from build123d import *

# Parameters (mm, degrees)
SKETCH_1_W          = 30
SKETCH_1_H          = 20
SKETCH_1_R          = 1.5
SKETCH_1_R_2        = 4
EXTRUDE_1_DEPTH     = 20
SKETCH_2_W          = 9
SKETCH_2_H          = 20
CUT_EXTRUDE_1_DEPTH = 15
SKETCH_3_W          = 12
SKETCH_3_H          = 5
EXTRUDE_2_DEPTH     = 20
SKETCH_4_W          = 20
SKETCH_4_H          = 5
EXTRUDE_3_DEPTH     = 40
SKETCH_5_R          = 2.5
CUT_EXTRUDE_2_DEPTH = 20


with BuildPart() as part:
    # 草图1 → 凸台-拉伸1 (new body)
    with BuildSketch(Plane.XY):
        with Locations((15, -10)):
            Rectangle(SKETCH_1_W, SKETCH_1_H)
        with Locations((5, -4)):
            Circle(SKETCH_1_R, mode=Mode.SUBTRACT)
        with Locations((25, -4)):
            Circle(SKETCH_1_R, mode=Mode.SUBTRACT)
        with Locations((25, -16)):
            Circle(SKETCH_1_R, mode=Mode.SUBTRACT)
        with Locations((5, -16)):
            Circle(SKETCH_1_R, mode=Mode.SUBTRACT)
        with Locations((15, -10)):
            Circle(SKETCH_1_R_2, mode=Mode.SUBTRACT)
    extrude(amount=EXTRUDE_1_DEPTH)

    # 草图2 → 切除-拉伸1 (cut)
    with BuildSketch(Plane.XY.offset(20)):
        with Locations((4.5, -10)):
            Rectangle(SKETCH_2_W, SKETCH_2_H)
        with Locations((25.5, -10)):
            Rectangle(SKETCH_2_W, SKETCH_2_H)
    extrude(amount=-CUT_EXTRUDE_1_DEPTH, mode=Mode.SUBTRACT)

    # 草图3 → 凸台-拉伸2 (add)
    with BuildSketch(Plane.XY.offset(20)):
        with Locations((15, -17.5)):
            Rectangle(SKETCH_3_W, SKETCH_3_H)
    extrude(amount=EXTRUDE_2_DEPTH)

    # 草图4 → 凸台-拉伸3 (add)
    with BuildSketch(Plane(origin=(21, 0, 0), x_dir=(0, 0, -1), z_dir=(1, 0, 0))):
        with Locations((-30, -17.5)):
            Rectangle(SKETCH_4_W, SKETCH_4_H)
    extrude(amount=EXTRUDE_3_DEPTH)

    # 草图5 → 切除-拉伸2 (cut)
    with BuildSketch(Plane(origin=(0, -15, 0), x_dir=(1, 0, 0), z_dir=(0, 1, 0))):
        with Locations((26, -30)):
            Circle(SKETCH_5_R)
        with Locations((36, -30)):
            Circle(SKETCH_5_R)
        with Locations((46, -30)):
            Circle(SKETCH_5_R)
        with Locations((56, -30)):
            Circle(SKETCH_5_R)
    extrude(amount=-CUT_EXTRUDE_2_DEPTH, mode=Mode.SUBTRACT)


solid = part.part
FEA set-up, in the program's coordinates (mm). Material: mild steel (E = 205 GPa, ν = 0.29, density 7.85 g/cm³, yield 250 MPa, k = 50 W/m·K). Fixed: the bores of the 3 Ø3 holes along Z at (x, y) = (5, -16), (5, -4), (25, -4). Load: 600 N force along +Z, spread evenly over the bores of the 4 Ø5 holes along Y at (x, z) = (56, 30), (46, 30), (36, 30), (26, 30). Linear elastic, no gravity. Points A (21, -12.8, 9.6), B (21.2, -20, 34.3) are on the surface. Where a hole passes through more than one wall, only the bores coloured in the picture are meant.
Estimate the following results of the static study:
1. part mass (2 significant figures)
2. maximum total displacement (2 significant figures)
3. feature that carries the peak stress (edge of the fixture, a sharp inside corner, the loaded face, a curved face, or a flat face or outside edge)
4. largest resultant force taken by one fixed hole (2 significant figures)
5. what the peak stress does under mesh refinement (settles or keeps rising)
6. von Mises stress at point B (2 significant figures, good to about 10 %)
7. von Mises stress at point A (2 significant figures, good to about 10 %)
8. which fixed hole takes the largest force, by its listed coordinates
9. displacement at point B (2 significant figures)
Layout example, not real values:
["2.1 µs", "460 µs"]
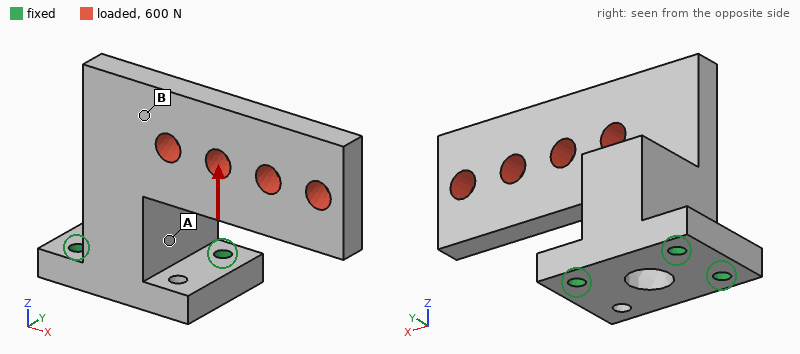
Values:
["81 g", "0.13 mm", "edge of the fixture", "1.2 kN", "keeps rising", "21 MPa", "55 MPa", "(25, -4)", "0.048 mm"]
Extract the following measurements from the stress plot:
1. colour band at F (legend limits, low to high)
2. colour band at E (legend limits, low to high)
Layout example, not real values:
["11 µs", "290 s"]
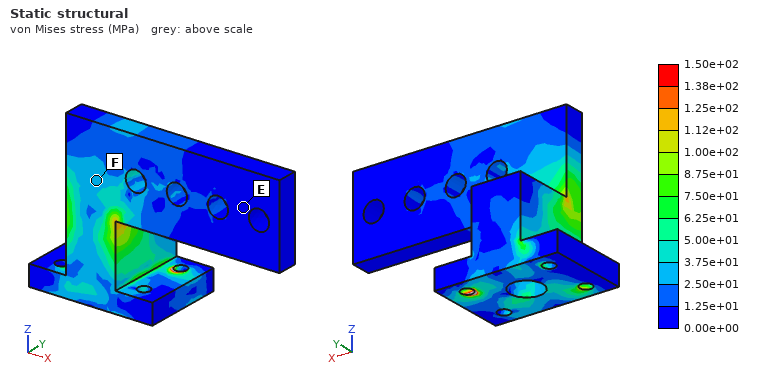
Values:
["2.50e+01 to 3.75e+01 MPa", "0.00e+00 to 1.25e+01 MPa"]
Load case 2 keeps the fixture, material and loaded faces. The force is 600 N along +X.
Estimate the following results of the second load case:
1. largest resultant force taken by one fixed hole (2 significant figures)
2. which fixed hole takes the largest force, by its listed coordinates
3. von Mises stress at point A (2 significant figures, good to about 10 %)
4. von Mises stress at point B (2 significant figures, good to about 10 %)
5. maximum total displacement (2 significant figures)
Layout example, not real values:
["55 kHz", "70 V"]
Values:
["1.0 kN", "(25, -4)", "44 MPa", "9.0 MPa", "69 µm"]
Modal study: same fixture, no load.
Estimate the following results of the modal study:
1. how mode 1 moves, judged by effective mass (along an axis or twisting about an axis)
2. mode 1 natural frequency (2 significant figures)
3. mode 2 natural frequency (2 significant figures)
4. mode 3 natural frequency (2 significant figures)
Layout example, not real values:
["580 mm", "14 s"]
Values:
["along Y", "1400 Hz", "2300 Hz", "4100 Hz"]
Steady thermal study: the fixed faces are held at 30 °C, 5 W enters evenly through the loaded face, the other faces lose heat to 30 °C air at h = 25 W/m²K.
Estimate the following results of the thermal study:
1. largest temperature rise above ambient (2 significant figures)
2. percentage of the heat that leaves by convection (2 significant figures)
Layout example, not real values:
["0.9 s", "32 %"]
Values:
["36 K", "40 %"]
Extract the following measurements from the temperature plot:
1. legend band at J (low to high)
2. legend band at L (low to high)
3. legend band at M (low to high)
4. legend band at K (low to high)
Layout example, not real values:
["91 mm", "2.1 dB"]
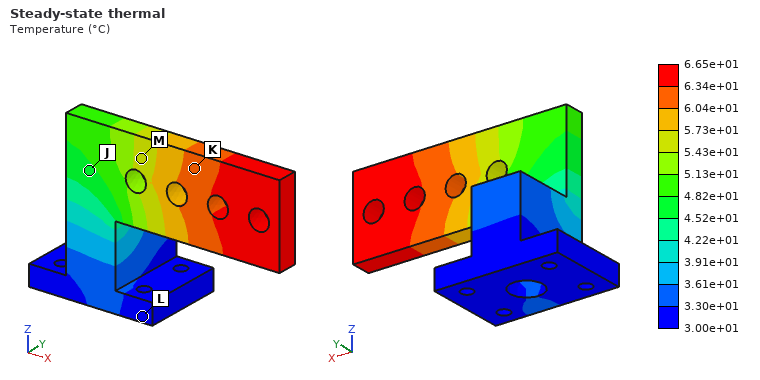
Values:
["4.52e+01 to 4.82e+01 °C", "3.00e+01 to 3.30e+01 °C", "5.43e+01 to 5.73e+01 °C", "6.04e+01 to 6.34e+01 °C"]
